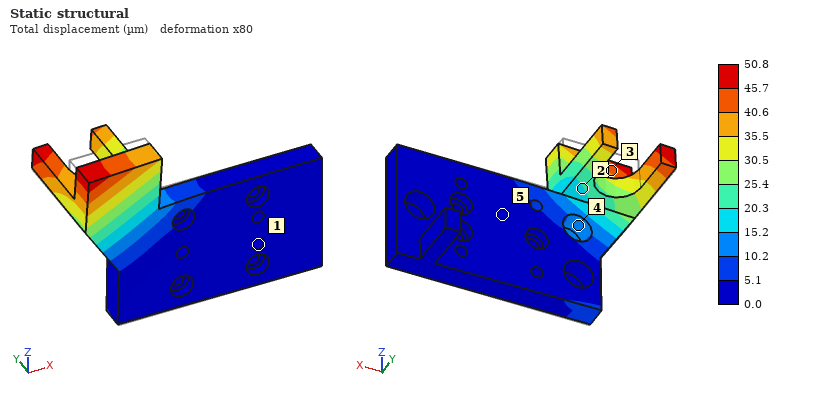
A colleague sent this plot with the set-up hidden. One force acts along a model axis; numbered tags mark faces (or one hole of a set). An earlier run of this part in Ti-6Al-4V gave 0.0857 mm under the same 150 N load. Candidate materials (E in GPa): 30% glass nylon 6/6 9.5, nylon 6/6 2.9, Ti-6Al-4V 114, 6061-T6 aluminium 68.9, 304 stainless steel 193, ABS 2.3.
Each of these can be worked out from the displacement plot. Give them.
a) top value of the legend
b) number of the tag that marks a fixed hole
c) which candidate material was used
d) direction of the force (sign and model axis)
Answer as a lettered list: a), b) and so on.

a) 50.8 µm
b) 1
c) 304 stainless steel
d) -Y
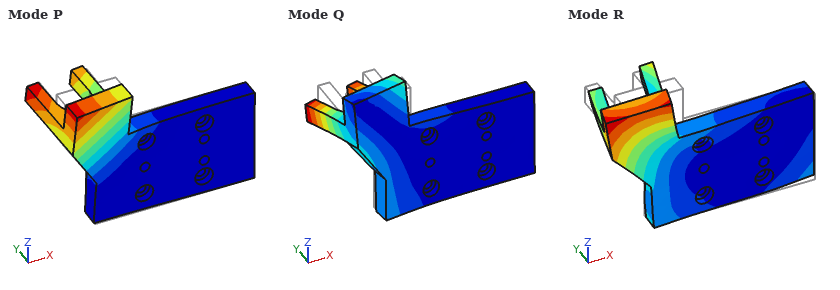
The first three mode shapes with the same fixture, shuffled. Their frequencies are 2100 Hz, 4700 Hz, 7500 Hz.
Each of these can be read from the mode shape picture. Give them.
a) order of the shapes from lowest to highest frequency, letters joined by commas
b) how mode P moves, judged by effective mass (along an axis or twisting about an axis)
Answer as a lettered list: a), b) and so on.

a) P, Q, R
b) along Y
